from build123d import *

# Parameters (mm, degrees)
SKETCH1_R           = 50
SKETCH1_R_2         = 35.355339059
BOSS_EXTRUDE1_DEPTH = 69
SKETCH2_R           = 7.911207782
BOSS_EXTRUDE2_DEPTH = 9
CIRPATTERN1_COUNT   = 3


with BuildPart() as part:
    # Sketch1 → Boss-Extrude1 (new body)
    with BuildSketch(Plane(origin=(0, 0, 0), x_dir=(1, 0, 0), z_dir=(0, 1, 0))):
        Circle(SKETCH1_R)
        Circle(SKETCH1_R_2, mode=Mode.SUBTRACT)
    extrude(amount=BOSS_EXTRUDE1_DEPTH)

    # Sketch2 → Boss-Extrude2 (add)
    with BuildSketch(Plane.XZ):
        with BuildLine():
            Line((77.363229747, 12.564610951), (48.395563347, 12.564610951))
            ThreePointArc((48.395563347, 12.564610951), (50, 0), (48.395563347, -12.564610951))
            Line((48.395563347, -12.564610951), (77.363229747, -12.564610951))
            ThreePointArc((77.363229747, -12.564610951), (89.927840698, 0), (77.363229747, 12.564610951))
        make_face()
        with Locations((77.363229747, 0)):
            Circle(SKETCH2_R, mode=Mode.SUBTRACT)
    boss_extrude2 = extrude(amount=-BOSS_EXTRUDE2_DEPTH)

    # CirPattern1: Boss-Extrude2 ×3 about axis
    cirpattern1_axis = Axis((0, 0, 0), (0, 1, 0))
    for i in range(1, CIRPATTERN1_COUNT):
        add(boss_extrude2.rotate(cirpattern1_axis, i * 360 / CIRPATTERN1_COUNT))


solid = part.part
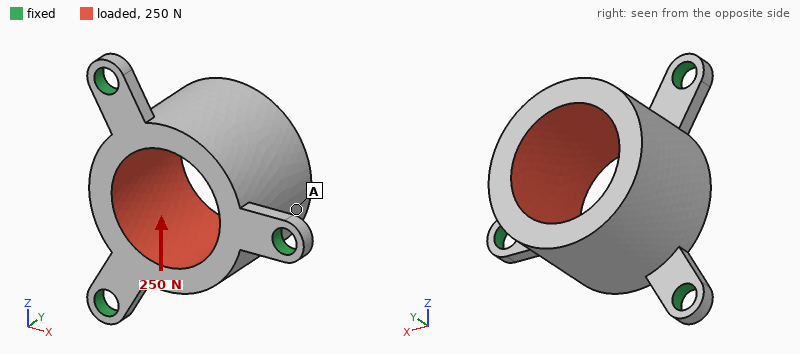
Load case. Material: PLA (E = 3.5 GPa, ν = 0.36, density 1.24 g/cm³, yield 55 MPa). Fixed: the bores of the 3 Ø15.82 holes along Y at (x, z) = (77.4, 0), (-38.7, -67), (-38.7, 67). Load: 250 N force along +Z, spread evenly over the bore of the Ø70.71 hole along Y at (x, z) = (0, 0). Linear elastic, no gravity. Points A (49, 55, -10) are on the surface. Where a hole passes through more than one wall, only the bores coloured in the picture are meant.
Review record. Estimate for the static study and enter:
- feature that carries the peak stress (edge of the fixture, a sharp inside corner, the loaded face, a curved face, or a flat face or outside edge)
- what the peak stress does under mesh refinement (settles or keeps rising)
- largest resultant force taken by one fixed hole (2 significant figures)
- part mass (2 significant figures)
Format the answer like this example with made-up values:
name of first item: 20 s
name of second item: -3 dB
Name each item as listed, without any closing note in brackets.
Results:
feature that carries the peak stress: edge of the fixture
what the peak stress does under mesh refinement: keeps rising
largest resultant force taken by one fixed hole: 120 N
part mass: 360 g
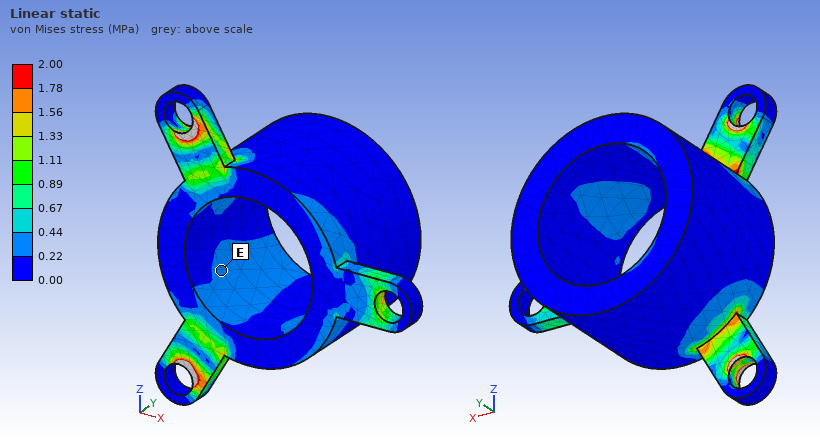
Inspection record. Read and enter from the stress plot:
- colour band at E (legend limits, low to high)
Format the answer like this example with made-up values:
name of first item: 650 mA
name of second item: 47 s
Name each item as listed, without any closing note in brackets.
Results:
colour band at E: 0.22 to 0.44 MPa
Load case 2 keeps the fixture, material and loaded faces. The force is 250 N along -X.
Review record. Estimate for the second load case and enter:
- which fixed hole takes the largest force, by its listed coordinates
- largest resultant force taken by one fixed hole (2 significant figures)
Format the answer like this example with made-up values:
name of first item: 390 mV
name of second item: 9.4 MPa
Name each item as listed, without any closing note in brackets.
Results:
which fixed hole takes the largest force, by its listed coordinates: (77.4, 0)
largest resultant force taken by one fixed hole: 140 N
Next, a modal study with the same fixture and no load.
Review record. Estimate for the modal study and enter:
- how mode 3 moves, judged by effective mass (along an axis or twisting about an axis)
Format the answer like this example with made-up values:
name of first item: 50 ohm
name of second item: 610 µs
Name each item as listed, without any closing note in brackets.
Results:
how mode 3 moves, judged by effective mass: along Y
